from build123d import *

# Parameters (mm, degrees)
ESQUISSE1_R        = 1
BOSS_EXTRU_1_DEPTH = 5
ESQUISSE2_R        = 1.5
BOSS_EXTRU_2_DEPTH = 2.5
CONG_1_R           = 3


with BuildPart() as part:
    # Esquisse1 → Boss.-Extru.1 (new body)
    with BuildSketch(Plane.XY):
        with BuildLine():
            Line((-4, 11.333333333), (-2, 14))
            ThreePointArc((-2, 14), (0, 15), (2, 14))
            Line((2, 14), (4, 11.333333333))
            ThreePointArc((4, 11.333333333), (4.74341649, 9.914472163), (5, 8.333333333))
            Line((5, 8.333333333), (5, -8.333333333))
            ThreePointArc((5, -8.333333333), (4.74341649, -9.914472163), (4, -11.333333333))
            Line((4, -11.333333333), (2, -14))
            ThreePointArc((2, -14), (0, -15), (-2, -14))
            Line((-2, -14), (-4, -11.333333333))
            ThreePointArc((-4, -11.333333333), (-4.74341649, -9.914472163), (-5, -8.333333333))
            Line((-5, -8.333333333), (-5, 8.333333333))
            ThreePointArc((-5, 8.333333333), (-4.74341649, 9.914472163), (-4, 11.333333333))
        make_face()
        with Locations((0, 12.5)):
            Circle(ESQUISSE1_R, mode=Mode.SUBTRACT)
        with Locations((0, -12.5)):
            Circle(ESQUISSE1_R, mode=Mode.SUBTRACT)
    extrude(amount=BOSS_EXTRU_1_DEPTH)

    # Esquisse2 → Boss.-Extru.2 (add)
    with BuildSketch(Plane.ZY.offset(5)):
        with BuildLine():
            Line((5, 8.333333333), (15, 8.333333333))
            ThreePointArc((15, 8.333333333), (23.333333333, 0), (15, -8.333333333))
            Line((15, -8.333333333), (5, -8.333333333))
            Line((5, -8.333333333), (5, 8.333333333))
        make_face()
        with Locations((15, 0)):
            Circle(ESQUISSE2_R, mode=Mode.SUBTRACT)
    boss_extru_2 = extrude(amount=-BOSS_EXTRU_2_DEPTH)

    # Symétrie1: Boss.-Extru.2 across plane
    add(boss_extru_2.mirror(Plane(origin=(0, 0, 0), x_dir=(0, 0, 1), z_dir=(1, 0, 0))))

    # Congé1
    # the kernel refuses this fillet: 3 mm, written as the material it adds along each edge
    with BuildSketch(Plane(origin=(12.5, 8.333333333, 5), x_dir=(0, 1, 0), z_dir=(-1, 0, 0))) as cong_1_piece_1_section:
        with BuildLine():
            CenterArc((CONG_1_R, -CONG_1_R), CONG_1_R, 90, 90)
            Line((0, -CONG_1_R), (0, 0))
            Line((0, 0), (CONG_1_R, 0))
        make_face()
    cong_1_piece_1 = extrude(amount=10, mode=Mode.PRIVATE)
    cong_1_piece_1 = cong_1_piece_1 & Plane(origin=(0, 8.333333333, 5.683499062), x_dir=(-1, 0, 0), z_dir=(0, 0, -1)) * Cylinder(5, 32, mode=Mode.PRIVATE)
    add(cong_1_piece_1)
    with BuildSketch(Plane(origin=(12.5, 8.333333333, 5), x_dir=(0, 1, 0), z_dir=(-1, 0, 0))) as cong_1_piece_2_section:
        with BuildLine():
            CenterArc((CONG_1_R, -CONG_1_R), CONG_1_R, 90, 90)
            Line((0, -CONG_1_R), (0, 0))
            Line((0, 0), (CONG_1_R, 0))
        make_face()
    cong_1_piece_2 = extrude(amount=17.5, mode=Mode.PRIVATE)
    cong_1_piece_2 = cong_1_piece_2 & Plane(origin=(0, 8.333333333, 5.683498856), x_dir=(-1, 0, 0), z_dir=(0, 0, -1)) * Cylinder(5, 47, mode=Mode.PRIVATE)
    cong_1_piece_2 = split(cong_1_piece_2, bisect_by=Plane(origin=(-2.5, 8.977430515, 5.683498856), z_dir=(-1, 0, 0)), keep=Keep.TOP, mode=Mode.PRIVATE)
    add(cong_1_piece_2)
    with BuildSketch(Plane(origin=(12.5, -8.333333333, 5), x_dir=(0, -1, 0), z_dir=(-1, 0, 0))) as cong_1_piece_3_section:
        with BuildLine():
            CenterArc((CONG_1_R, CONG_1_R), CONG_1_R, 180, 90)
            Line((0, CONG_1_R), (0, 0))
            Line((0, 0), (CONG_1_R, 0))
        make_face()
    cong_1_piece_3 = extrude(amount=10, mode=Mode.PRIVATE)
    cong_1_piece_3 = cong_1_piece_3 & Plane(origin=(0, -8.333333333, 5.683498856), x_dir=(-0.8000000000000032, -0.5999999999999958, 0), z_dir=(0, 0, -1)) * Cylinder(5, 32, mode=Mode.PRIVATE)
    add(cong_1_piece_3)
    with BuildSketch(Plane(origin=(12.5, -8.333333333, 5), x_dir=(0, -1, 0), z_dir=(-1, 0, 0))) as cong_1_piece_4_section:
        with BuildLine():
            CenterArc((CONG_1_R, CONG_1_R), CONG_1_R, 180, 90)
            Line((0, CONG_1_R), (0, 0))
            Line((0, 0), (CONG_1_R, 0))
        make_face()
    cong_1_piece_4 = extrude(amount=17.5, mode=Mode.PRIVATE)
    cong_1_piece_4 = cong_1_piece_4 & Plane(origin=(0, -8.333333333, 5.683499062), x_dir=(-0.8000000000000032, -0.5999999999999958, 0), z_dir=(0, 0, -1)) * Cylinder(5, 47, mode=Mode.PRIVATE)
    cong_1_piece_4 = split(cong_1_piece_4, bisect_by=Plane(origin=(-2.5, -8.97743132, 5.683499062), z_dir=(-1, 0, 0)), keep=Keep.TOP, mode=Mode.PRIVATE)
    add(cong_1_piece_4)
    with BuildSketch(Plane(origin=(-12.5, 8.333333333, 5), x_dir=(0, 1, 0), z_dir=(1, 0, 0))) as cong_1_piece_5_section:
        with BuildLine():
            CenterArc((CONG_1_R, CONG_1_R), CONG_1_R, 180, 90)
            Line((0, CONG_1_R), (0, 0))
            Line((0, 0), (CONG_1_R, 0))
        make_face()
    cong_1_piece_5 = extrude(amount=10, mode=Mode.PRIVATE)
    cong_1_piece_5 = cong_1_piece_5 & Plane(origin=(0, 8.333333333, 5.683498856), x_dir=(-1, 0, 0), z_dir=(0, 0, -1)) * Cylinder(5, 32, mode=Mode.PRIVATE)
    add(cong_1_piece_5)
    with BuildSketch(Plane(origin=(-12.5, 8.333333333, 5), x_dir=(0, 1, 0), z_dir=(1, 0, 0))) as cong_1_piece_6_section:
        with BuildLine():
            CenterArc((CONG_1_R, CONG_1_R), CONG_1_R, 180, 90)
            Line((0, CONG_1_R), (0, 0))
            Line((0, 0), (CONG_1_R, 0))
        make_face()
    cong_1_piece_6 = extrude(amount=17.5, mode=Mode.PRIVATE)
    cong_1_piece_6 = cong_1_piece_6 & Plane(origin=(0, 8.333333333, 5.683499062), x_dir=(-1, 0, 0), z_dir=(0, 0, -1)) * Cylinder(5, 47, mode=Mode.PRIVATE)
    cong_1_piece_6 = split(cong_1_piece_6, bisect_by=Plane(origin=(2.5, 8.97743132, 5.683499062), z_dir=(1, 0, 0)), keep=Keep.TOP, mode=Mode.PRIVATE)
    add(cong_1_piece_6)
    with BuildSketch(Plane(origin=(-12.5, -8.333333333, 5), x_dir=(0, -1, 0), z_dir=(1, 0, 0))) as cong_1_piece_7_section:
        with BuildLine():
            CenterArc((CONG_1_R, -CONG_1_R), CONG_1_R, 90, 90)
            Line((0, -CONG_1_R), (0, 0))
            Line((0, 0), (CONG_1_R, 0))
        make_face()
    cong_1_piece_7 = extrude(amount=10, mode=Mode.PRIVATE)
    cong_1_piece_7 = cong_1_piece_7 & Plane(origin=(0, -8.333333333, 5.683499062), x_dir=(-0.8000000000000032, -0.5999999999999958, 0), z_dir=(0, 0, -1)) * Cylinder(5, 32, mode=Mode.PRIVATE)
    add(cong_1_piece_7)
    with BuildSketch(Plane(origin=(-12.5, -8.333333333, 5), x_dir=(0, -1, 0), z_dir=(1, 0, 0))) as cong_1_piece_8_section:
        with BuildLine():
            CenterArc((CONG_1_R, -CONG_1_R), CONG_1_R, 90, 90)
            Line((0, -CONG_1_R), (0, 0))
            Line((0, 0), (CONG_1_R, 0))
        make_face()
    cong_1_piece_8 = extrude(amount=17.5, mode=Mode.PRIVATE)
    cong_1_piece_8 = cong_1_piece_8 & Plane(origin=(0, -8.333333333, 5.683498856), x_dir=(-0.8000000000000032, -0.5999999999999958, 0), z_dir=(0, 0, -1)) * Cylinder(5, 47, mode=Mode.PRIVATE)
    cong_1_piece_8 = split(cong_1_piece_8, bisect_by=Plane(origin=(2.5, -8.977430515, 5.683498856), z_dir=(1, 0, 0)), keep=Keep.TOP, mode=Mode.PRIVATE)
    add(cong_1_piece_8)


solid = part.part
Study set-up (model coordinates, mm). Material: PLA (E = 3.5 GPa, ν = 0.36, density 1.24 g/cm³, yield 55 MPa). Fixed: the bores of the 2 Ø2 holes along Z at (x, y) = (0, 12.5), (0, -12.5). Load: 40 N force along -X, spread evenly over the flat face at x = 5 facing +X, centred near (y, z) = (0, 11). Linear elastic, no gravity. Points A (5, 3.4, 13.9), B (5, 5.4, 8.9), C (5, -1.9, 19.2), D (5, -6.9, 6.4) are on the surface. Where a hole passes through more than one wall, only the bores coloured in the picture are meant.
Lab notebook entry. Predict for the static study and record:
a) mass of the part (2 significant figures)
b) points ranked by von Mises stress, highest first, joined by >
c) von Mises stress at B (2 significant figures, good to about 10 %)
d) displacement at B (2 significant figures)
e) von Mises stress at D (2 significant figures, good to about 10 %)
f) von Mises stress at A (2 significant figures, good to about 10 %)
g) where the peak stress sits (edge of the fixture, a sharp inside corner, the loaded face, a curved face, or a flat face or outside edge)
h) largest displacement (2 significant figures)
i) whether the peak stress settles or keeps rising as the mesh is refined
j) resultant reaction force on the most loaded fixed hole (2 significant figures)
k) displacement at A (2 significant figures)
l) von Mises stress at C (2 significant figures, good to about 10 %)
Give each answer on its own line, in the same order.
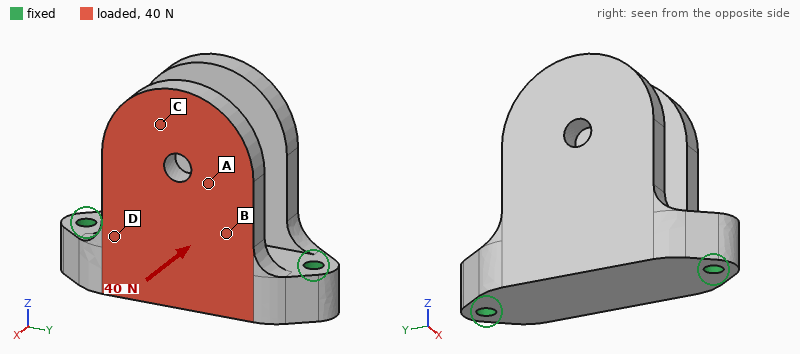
3.3 g
D > B > A > C
8.4 MPa
0.075 mm
12 MPa
3.9 MPa
edge of the fixture
0.41 mm
keeps rising
20 N
0.18 mm
1.2 MPa
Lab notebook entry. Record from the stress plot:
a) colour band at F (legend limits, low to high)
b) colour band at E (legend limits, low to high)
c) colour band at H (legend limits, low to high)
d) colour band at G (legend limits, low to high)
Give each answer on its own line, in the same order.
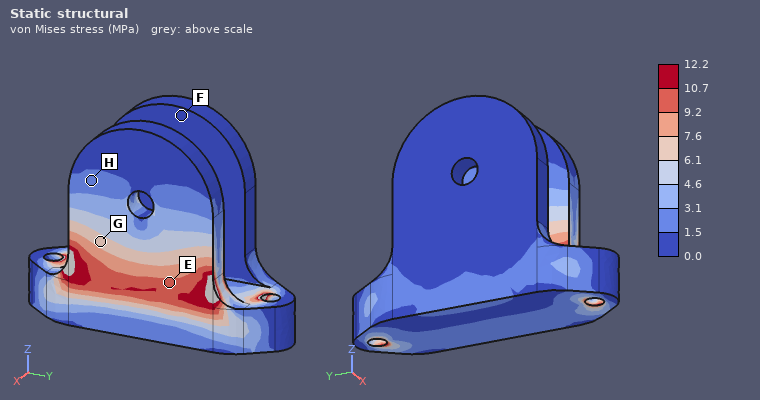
0.0 to 1.5 MPa
9.2 to 10.7 MPa
1.5 to 3.1 MPa
6.1 to 7.6 MPa
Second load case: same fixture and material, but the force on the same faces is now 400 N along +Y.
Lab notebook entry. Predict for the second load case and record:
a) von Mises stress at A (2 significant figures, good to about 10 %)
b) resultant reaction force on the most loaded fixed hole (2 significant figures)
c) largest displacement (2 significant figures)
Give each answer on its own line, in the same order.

19 MPa
260 N
0.25 mm
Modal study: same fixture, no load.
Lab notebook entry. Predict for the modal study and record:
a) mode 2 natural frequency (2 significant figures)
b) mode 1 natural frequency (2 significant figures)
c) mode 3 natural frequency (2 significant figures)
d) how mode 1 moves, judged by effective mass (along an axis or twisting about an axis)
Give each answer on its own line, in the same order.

2100 Hz
1800 Hz
5500 Hz
along X
